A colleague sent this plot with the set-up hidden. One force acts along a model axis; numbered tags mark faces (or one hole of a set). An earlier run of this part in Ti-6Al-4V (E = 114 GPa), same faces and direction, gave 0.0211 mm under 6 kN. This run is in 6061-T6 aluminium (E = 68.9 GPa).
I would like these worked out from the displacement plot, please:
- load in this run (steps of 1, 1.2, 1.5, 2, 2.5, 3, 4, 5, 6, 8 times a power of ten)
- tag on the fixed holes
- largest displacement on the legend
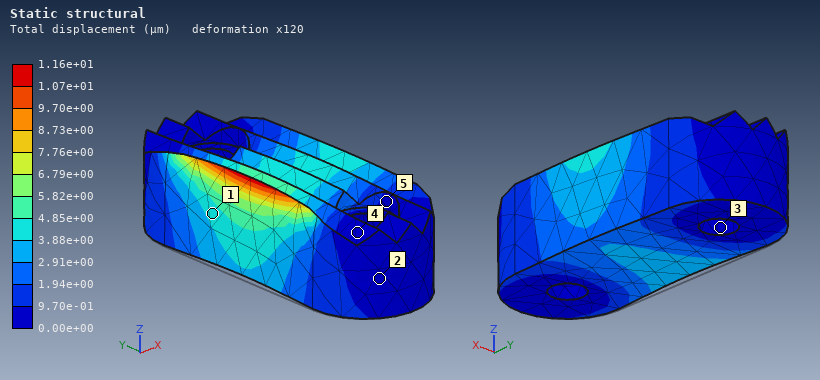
2 kN
3
1.16e+01 µm
